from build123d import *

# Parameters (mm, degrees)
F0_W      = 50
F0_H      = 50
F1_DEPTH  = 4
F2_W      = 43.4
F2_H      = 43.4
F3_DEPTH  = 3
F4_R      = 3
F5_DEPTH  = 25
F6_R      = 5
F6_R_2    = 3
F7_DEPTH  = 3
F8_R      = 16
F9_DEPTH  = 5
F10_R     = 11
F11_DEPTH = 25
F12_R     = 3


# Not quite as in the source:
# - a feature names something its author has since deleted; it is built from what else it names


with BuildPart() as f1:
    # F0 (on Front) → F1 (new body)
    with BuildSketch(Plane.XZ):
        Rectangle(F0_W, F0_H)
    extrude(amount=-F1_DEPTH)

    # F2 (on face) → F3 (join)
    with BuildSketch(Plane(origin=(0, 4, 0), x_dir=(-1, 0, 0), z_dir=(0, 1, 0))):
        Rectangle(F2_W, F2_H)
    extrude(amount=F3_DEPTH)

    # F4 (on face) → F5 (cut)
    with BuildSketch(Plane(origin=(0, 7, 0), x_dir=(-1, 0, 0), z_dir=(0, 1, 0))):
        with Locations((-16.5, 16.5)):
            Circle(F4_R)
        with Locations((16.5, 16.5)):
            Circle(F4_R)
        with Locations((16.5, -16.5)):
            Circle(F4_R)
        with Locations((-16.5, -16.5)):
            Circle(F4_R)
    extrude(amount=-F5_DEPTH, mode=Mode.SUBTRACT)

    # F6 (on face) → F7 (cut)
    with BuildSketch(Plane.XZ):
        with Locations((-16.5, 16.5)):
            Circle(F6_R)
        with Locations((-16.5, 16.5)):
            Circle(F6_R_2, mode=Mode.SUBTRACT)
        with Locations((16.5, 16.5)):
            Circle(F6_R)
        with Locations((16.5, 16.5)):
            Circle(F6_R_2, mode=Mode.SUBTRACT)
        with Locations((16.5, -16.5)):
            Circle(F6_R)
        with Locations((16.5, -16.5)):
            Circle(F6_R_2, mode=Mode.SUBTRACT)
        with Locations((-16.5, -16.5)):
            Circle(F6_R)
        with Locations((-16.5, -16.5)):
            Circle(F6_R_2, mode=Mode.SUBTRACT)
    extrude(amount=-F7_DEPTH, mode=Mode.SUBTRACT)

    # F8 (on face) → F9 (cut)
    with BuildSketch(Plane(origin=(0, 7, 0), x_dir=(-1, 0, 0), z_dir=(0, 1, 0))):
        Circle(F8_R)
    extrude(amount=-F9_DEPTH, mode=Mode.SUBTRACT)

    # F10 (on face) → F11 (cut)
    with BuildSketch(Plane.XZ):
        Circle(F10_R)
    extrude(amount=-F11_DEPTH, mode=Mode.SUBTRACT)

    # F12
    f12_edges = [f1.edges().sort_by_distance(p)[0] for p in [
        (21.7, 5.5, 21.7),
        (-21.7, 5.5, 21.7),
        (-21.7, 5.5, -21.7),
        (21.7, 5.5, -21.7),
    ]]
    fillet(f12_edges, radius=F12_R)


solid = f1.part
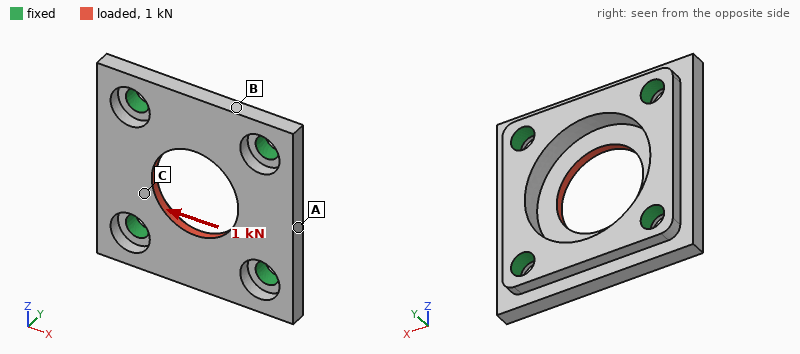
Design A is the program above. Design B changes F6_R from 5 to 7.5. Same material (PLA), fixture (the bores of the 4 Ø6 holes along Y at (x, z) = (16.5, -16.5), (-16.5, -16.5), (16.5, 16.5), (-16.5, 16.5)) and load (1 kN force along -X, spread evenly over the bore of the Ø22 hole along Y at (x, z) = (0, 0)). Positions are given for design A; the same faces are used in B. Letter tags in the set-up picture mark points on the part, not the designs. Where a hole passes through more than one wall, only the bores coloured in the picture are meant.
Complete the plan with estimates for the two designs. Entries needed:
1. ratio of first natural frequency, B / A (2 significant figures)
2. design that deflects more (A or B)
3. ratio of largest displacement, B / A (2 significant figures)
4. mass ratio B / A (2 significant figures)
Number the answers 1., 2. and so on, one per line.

1. 0.93
2. B
3. 1.3
4. 0.88
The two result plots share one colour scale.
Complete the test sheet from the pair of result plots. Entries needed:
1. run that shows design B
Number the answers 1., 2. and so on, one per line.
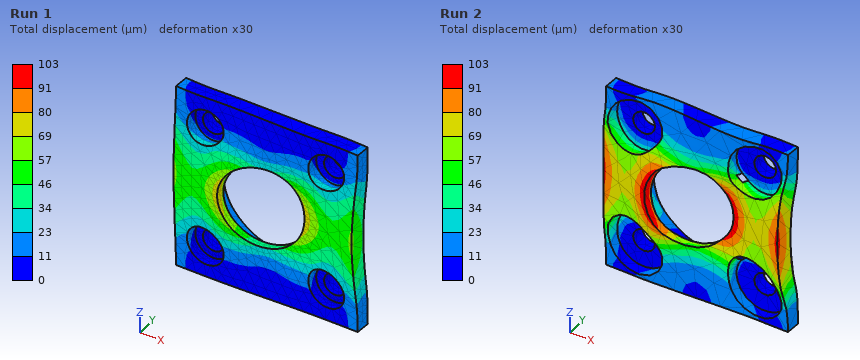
1. Run 2
